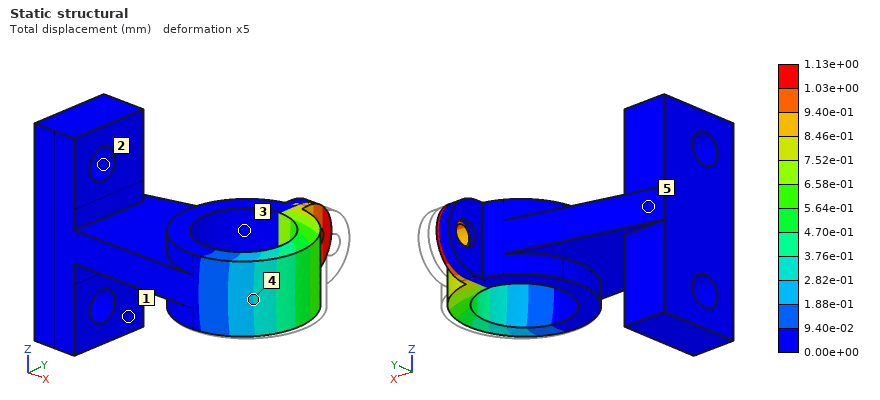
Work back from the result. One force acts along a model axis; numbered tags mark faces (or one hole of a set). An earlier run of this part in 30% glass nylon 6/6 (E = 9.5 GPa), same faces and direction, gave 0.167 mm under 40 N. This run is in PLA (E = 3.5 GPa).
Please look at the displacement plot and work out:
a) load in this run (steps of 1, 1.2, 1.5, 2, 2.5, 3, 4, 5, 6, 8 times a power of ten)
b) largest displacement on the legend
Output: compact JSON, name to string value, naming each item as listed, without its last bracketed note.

{"load in this run": "100 N", "largest displacement on the legend": "1.13e+00 mm"}
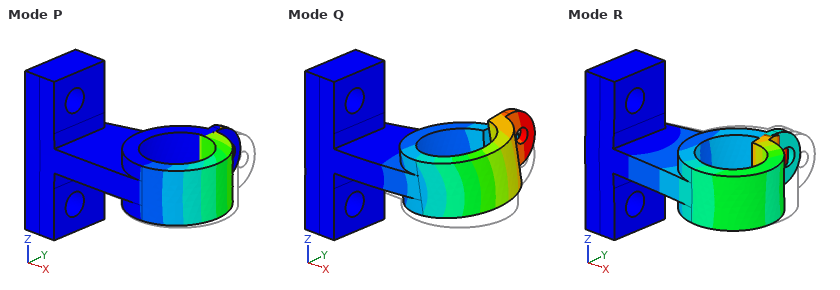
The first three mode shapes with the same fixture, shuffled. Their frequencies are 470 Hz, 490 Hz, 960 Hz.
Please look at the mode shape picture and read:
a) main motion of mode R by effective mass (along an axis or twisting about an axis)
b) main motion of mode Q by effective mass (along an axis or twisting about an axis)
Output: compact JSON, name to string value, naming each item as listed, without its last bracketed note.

{"main motion of mode R by effective mass": "along Y", "main motion of mode Q by effective mass": "along Z"}
